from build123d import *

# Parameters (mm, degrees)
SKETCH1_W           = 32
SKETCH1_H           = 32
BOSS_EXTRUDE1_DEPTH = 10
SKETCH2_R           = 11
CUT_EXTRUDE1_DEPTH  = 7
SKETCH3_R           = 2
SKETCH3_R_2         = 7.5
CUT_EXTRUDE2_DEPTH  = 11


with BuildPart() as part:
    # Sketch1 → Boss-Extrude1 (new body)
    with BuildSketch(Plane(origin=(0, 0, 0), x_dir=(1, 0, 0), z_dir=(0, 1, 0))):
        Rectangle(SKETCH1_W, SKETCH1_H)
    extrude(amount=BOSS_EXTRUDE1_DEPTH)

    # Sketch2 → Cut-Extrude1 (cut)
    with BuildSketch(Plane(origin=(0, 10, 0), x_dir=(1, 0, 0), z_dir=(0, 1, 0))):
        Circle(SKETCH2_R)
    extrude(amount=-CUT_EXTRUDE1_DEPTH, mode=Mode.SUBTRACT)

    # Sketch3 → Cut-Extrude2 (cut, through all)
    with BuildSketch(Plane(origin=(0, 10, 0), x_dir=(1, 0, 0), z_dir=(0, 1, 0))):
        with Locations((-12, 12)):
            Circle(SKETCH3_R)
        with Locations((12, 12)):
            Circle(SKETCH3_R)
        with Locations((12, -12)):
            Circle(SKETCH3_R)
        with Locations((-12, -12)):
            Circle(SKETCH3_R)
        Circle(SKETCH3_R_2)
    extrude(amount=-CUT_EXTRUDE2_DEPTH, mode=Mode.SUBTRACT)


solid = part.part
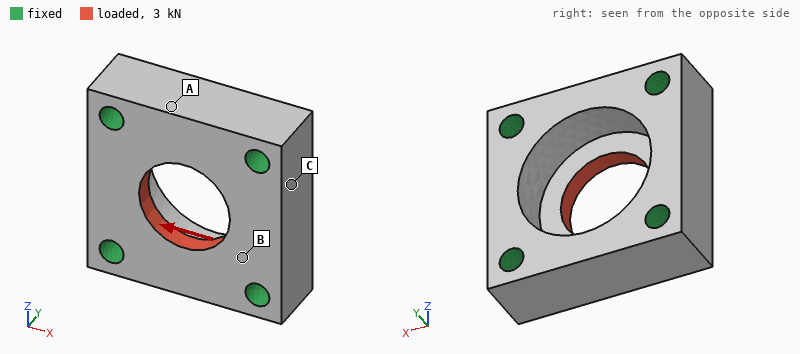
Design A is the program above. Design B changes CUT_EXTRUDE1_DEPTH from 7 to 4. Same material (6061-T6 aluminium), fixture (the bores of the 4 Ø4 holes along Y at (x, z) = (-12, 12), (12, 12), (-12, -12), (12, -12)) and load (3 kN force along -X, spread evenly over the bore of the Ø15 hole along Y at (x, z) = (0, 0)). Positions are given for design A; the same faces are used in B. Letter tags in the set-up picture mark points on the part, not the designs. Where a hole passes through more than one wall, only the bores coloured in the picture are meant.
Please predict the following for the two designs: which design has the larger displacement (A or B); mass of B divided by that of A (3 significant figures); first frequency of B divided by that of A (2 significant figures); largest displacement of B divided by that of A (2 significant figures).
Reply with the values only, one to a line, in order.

A
1.09
1.00
0.59
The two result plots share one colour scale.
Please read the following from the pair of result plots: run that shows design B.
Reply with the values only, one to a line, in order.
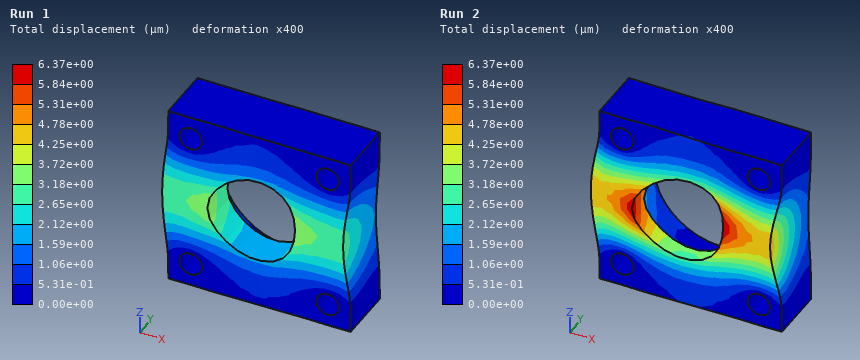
Run 1
